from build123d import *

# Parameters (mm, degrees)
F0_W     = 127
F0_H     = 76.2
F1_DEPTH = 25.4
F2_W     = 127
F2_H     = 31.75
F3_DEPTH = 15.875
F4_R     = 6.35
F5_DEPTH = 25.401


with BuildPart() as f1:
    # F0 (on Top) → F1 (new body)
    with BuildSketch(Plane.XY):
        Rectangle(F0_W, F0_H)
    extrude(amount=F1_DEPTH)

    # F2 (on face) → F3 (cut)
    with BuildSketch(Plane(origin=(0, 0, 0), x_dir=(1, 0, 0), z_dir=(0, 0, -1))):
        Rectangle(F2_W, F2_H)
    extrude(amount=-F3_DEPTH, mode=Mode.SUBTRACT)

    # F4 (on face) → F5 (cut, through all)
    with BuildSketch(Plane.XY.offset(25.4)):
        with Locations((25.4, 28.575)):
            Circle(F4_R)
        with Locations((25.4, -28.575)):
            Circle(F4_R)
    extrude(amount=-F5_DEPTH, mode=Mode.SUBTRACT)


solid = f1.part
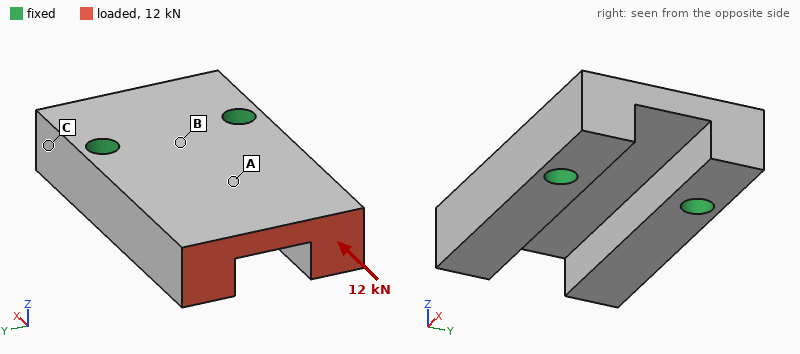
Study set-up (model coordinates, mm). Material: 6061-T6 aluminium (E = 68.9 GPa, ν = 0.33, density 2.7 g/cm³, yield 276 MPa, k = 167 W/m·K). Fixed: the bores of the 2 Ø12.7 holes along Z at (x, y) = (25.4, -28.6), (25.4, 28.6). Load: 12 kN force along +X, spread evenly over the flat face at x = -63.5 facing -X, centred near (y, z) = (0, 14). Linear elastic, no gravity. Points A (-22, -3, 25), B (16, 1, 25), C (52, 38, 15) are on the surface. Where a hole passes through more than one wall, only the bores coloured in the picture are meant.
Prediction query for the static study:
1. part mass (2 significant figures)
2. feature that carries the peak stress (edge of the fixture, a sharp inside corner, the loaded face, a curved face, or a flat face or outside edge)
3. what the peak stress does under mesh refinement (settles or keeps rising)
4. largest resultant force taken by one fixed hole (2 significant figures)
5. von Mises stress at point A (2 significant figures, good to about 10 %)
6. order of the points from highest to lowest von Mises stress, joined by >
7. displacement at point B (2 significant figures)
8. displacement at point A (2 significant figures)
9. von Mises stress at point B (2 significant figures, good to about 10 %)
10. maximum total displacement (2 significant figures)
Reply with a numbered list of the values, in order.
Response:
1. 470 g
2. edge of the fixture
3. keeps rising
4. 6.0 kN
5. 7.9 MPa
6. A > B > C
7. 2.8 µm
8. 6.6 µm
9. 3.9 MPa
10. 12 µm
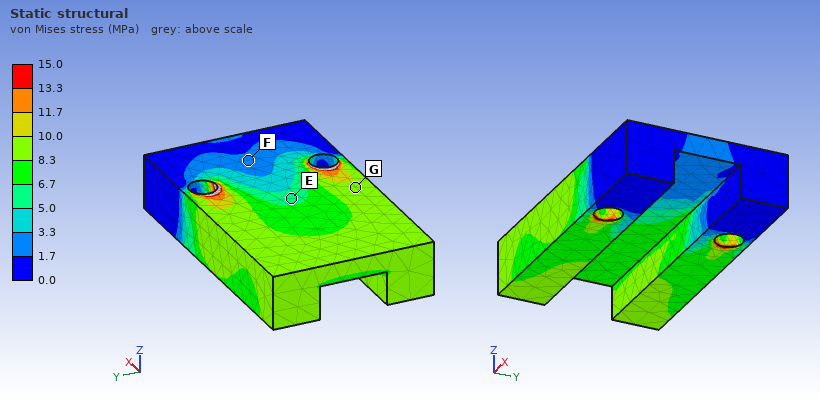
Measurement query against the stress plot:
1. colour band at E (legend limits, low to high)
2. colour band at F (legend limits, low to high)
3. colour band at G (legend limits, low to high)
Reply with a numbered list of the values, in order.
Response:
1. 5.0 to 6.7 MPa
2. 1.7 to 3.3 MPa
3. 8.3 to 10.0 MPa
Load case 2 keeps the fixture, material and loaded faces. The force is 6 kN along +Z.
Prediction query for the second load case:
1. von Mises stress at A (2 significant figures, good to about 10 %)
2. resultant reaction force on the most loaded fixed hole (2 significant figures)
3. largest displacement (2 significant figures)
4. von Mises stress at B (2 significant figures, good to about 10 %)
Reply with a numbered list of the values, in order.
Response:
1. 31 MPa
2. 3.2 kN
3. 0.28 mm
4. 36 MPa
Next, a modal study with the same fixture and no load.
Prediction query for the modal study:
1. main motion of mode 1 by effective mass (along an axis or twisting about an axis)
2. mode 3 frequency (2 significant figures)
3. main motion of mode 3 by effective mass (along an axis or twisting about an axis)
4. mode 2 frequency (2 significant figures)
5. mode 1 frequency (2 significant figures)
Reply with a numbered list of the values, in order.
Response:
1. along Z
2. 5800 Hz
3. along Y
4. 3700 Hz
5. 2600 Hz
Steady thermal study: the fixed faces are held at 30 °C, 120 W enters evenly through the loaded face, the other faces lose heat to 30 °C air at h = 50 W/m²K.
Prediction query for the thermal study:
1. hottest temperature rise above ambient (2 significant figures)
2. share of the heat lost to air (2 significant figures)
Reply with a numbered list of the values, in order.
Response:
1. 39 K
2. 16 %
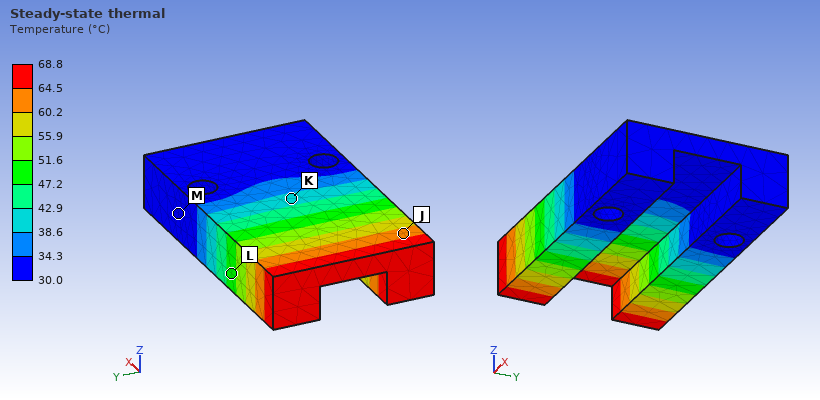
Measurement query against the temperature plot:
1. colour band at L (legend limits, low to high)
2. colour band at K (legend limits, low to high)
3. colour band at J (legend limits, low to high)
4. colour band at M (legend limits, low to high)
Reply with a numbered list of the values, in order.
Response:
1. 47.2 to 51.6 °C
2. 38.6 to 42.9 °C
3. 60.2 to 64.5 °C
4. 30.0 to 34.3 °C
